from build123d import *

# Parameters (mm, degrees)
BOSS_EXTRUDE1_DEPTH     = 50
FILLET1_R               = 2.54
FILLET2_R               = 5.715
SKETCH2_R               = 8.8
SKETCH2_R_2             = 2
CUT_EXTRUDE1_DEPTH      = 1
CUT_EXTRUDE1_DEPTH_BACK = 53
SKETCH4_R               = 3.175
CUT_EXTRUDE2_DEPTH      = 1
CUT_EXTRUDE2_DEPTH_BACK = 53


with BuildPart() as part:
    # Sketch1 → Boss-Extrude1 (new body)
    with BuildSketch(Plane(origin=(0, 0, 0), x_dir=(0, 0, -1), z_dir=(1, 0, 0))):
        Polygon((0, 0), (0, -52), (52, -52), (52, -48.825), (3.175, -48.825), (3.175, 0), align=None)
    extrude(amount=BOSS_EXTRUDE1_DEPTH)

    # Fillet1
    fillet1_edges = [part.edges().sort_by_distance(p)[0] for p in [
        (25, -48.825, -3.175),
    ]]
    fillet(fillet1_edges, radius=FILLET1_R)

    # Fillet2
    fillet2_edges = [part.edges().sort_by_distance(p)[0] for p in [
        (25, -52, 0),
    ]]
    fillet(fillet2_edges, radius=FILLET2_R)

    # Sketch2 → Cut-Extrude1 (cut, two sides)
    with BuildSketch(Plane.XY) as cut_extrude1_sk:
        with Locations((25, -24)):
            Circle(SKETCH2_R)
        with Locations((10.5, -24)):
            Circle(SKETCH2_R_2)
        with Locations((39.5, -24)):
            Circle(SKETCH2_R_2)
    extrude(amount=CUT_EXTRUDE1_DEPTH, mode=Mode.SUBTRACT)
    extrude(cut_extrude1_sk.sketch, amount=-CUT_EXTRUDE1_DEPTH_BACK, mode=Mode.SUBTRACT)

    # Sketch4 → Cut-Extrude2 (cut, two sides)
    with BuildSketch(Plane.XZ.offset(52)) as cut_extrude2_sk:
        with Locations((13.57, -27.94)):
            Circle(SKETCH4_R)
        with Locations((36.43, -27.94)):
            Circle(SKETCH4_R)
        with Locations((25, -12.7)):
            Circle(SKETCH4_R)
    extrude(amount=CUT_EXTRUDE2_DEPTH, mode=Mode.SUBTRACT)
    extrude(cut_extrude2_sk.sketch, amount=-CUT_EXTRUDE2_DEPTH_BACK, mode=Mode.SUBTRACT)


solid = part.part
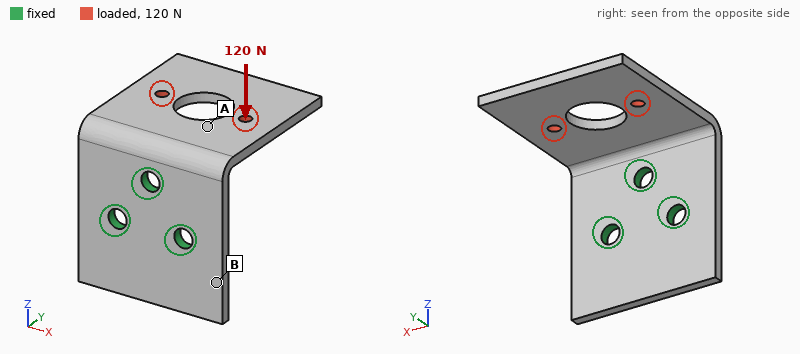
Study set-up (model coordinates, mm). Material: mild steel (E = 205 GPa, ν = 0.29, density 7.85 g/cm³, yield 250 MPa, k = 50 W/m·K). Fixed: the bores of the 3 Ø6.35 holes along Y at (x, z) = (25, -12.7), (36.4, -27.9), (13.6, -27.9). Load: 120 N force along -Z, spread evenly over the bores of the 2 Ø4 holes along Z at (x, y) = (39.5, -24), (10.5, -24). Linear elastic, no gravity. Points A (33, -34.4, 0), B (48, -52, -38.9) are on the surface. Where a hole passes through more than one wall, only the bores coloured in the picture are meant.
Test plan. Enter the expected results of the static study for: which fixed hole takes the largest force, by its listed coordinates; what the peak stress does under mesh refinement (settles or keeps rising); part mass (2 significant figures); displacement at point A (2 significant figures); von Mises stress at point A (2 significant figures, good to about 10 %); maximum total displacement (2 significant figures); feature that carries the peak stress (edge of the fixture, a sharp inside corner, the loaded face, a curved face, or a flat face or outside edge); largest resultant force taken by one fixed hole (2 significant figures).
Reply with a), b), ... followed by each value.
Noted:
a) (25, -12.7)
b) keeps rising
c) 110 g
d) 0.030 mm
e) 17 MPa
f) 0.12 mm
g) edge of the fixture
h) 120 N
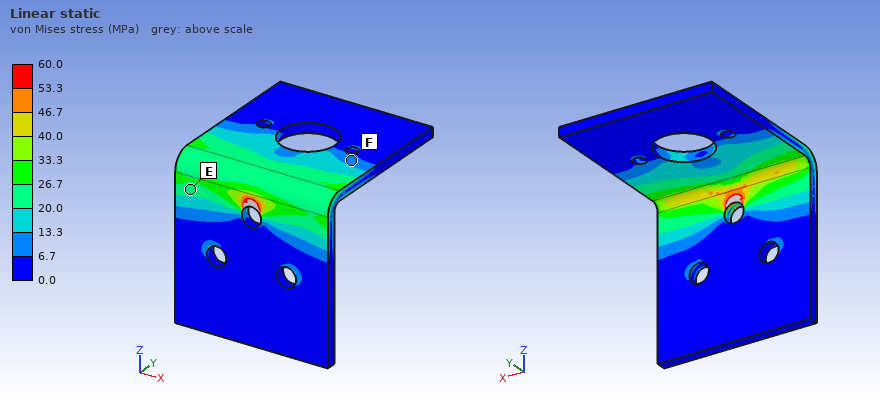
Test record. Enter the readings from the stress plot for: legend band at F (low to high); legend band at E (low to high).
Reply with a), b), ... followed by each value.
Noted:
a) 6.7 to 13.3 MPa
b) 20.0 to 26.7 MPa
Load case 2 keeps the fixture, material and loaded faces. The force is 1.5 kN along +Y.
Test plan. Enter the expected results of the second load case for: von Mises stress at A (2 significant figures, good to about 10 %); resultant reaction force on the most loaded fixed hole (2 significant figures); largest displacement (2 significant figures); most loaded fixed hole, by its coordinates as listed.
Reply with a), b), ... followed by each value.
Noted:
a) 27 MPa
b) 1.8 kN
c) 0.18 mm
d) (25, -12.7)
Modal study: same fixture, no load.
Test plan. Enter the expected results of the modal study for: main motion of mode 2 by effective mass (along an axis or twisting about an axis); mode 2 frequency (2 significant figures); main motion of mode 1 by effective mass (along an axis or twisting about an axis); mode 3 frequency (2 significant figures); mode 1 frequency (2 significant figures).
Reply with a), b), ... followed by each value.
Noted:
a) along X
b) 1400 Hz
c) along Z
d) 2300 Hz
e) 790 Hz
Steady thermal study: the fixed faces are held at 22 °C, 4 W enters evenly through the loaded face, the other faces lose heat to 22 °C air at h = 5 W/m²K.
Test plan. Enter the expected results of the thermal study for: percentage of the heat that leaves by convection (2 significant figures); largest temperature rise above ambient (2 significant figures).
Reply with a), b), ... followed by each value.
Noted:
a) 11 %
b) 23 K
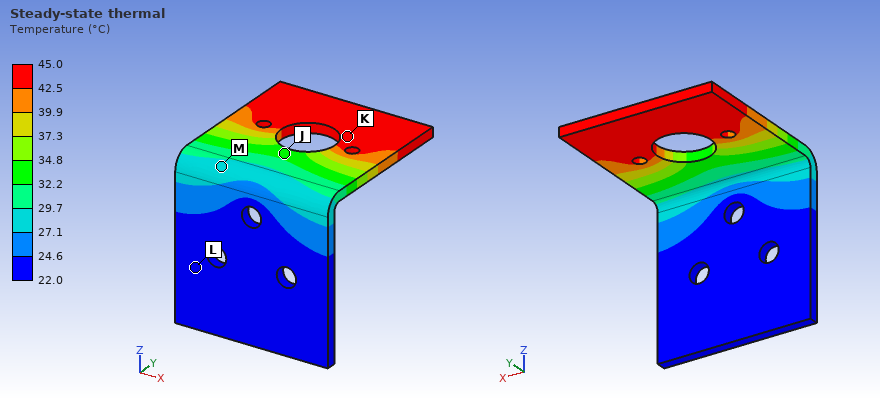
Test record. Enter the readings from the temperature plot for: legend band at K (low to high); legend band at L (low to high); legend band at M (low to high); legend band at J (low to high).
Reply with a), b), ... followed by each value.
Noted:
a) 42.5 to 45.0 °C
b) 22.0 to 24.6 °C
c) 27.1 to 29.7 °C
d) 32.2 to 34.8 °C
